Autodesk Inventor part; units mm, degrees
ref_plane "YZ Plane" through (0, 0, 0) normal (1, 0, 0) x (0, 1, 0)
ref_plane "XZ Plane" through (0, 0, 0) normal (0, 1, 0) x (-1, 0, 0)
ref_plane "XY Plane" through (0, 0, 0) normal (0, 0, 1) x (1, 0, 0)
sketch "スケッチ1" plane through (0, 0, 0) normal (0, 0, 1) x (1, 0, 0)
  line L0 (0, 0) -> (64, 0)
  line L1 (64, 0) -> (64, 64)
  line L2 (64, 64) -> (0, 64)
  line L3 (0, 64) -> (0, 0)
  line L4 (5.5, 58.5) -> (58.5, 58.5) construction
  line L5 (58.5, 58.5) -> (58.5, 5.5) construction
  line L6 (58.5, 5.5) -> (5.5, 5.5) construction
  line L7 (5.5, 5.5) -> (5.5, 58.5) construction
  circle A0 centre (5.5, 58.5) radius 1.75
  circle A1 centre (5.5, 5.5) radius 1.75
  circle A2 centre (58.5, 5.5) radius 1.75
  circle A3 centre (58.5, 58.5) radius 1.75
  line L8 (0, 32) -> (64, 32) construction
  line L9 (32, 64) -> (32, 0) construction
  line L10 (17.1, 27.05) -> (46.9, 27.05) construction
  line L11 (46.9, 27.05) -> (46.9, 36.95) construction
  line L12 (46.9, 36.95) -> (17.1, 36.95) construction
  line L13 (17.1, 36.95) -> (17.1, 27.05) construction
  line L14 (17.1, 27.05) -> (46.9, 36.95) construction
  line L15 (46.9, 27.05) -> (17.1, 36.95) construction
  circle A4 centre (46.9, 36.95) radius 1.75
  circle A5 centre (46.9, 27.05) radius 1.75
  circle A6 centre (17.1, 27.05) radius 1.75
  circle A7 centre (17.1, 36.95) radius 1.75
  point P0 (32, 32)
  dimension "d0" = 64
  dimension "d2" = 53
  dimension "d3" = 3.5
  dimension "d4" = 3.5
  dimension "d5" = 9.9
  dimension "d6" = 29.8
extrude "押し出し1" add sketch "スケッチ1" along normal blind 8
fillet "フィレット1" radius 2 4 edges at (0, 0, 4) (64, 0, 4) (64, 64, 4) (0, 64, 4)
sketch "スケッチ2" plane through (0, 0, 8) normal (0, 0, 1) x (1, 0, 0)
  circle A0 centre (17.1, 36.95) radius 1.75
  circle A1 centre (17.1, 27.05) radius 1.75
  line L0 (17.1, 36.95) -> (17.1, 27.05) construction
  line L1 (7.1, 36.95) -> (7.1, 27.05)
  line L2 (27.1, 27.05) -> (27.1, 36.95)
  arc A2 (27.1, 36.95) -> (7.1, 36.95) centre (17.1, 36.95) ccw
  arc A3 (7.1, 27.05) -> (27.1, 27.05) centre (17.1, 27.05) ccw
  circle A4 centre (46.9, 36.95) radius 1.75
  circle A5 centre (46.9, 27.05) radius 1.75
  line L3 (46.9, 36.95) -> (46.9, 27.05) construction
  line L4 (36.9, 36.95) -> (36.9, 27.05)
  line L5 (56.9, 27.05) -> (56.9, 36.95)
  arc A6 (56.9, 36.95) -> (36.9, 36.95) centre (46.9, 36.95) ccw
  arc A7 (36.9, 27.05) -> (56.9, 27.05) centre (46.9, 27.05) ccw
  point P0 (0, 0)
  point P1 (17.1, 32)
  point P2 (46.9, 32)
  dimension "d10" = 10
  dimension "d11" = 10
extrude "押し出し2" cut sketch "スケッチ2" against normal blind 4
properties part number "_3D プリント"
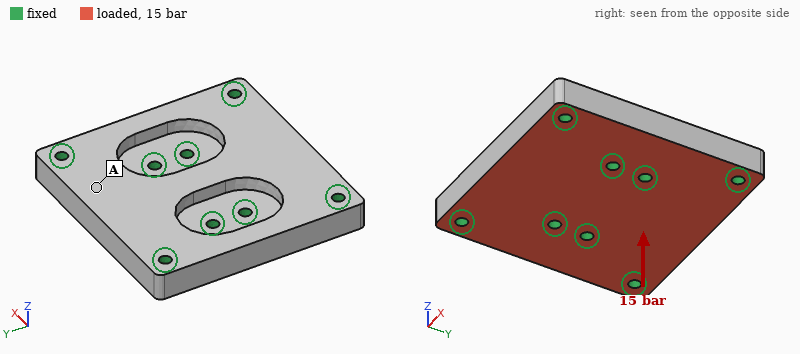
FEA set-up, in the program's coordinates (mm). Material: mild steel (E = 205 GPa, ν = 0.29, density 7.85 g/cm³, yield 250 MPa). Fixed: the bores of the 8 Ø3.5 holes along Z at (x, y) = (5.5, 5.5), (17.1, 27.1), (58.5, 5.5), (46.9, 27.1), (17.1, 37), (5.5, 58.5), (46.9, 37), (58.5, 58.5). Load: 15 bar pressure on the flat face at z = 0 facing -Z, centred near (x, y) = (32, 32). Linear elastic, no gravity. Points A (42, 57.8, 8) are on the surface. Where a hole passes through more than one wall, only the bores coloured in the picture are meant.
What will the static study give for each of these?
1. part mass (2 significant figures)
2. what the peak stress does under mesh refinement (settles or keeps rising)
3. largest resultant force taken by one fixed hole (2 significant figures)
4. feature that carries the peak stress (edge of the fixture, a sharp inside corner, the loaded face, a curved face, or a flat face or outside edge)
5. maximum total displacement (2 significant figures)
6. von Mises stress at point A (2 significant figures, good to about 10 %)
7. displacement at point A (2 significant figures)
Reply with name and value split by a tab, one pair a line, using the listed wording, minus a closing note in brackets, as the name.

part mass	220 g
what the peak stress does under mesh refinement	keeps rising
largest resultant force taken by one fixed hole	810 N
feature that carries the peak stress	edge of the fixture
maximum total displacement	4.3 µm
von Mises stress at point A	9.0 MPa
displacement at point A	3.0 µm
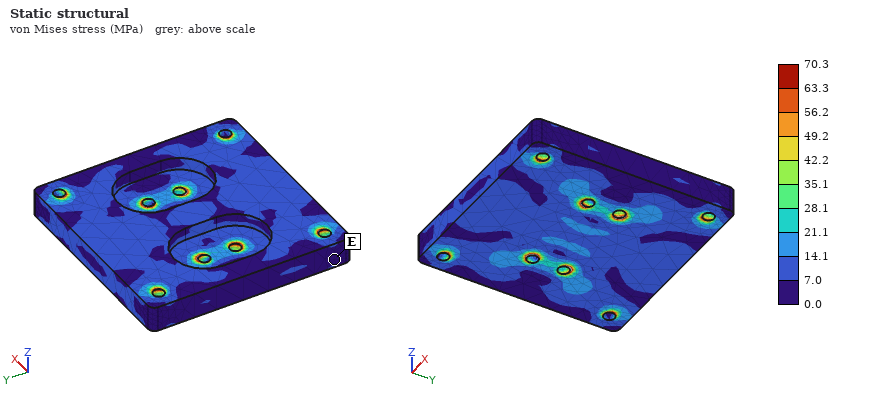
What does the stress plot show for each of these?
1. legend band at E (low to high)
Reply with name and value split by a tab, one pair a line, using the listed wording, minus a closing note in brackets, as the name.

legend band at E	0.0 to 7.0 MPa
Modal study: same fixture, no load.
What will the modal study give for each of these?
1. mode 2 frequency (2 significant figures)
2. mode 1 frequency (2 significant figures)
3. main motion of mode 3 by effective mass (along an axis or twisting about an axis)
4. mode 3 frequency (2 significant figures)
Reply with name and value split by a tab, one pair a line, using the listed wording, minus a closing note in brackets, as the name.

mode 2 frequency	14 kHz
mode 1 frequency	14 kHz
main motion of mode 3 by effective mass	twisting about Y
mode 3 frequency	20 kHz
